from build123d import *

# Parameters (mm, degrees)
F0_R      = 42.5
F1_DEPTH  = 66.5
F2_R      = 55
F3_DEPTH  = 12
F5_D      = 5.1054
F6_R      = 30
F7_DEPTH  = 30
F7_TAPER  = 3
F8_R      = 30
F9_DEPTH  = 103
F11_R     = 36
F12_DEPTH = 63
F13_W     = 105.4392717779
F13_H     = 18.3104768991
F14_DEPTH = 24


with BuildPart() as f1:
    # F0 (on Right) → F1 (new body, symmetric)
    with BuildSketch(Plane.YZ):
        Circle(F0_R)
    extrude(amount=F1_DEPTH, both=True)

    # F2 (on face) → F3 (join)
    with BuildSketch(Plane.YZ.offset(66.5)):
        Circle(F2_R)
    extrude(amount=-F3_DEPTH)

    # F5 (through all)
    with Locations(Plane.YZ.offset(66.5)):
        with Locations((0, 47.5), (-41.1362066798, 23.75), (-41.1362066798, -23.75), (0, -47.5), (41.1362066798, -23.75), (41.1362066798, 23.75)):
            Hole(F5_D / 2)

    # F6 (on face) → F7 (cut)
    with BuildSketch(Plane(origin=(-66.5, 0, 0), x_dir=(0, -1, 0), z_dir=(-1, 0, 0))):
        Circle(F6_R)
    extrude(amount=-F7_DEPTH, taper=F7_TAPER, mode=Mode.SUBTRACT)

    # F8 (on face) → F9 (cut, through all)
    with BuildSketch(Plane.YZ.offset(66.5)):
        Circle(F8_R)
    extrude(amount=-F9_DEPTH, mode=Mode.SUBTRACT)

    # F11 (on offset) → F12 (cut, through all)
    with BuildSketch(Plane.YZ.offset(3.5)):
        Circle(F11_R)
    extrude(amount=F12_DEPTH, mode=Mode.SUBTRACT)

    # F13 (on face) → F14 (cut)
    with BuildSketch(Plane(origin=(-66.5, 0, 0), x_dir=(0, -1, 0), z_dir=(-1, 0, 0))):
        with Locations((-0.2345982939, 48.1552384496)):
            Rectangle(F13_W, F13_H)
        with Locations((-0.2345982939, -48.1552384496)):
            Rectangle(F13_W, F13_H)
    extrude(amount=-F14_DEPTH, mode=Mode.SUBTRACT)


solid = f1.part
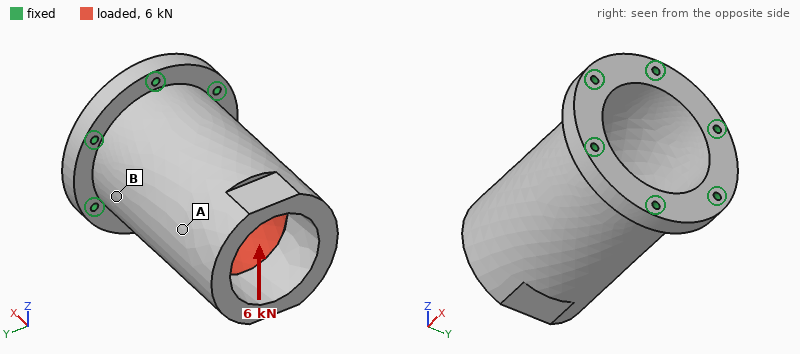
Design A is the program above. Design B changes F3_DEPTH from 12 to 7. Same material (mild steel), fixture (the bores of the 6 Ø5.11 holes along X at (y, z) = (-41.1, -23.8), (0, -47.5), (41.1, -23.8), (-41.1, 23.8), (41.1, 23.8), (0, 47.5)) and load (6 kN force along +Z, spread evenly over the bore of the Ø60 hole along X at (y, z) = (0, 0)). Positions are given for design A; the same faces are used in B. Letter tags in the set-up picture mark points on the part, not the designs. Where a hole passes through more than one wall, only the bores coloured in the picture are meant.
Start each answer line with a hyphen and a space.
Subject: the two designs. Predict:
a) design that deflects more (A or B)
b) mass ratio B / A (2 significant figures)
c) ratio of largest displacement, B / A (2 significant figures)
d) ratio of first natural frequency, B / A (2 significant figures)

- B
- 0.95
- 1.5
- 0.82
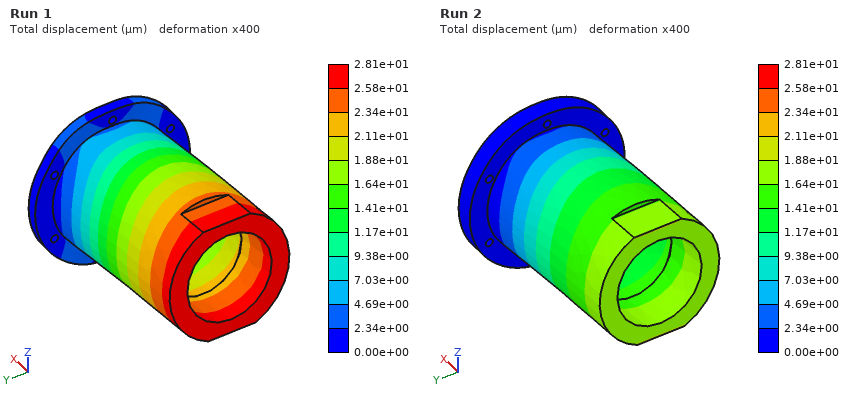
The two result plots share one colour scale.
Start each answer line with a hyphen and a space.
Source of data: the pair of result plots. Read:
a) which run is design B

- Run 1
